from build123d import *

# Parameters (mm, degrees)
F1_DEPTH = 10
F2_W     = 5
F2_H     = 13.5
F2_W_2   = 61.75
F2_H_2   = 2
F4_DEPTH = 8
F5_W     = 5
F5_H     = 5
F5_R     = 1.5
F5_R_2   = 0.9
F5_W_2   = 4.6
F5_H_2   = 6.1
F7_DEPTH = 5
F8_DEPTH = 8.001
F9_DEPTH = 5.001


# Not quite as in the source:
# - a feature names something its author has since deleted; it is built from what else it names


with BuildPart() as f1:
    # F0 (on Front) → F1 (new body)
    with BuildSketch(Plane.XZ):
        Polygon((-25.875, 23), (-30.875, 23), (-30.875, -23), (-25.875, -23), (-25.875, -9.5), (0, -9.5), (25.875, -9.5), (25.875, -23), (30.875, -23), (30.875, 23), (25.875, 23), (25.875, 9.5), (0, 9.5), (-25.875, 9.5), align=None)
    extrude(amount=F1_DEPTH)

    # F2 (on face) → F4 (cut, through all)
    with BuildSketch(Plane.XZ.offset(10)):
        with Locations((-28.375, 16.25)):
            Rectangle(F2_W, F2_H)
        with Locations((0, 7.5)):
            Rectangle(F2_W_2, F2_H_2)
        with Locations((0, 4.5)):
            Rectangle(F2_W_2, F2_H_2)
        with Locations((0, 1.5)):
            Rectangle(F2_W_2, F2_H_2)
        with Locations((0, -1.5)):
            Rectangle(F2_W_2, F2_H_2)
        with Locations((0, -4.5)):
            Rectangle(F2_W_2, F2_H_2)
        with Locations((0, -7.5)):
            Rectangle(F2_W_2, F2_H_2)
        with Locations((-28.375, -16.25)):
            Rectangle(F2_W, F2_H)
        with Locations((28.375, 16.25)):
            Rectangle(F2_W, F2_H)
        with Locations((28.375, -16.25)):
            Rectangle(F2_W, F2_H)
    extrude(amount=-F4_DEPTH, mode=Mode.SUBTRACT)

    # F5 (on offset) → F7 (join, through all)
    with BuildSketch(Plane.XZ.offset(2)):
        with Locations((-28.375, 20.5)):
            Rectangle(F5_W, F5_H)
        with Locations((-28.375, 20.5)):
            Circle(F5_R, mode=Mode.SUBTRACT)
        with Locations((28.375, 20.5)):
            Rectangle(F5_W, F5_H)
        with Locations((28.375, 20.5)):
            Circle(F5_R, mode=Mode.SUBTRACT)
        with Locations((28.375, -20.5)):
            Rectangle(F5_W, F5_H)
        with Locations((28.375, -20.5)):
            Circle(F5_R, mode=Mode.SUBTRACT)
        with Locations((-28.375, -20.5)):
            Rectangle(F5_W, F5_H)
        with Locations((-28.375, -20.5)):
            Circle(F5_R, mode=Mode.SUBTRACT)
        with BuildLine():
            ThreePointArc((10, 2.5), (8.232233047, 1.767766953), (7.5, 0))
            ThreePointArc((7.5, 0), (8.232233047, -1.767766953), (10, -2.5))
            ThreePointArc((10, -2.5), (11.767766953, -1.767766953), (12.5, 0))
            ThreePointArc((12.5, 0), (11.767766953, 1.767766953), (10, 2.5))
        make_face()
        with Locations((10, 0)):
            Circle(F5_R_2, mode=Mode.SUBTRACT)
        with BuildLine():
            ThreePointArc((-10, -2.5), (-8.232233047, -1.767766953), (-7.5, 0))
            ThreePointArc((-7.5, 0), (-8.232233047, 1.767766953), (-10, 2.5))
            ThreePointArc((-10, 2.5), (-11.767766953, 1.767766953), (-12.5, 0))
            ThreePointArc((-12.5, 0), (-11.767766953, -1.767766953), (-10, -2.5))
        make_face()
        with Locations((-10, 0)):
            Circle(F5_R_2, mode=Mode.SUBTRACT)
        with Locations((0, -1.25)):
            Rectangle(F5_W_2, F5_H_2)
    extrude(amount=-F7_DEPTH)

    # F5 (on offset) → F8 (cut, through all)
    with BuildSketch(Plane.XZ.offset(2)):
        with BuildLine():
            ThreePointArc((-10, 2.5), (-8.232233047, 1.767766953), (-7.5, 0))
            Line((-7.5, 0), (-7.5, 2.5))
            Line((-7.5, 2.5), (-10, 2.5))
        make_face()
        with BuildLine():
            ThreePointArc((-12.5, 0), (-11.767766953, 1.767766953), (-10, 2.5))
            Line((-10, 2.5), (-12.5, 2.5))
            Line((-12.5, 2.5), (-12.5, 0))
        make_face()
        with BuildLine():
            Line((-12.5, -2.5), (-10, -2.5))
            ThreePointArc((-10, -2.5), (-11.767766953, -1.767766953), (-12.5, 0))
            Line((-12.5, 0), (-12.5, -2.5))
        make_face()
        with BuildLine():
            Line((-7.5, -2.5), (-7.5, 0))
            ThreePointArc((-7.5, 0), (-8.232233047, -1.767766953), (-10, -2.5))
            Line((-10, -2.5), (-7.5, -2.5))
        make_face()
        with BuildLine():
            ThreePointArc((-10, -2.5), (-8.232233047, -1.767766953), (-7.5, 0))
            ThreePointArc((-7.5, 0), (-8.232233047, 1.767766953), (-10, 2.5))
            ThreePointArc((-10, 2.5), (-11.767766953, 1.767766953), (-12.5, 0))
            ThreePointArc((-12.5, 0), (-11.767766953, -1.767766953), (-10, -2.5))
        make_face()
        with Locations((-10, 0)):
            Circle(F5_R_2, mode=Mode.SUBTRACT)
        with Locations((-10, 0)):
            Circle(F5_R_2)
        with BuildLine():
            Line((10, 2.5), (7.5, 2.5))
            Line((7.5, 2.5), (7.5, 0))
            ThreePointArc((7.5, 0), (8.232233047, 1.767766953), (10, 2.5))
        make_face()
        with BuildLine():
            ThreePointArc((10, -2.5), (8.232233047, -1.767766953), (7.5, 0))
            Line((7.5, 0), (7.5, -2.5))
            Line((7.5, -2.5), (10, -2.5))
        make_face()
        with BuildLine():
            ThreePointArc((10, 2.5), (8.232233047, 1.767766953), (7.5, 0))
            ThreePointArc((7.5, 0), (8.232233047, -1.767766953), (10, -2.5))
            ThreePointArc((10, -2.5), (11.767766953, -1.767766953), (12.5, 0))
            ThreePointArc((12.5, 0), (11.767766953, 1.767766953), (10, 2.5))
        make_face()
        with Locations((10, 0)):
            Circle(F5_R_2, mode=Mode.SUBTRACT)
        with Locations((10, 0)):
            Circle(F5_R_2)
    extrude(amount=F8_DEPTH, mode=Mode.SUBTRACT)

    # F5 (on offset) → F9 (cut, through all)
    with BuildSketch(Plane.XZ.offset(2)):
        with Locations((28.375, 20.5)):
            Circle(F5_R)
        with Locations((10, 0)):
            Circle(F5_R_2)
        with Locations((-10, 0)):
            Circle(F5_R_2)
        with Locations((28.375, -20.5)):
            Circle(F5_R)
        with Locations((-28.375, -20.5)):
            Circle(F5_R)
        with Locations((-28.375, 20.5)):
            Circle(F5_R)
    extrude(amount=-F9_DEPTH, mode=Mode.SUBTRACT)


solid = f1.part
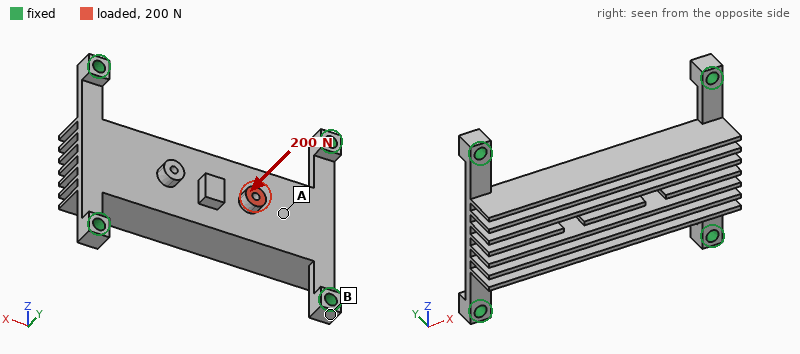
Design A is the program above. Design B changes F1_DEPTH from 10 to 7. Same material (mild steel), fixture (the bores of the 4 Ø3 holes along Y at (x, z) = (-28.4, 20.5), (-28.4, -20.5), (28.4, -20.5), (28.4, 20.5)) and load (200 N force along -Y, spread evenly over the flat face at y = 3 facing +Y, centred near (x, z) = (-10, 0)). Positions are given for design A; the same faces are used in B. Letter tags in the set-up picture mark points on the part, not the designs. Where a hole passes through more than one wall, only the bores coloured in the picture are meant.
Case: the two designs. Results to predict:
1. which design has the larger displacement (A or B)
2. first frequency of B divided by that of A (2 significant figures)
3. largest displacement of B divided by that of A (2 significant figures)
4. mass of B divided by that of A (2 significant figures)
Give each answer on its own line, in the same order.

B
1.0
1.2
0.81
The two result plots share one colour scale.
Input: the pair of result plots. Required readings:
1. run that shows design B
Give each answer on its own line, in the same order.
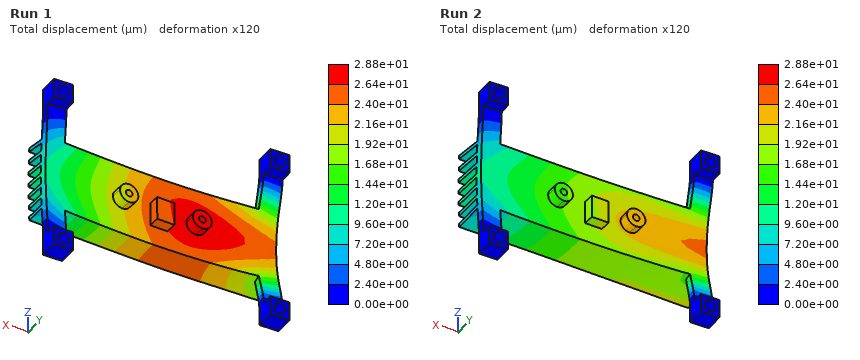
Run 1
